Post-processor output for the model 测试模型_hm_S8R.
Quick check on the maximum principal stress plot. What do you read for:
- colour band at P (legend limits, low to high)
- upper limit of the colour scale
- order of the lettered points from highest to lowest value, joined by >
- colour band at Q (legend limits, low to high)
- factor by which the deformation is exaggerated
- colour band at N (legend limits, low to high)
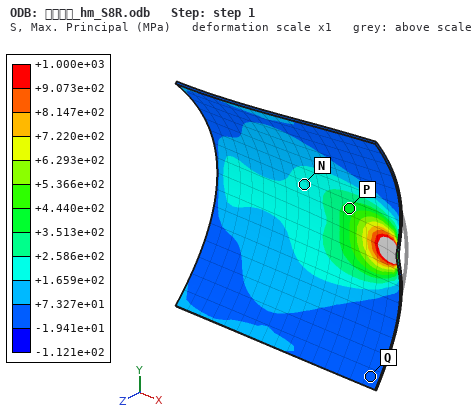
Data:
+3.513e+02 to +4.440e+02 MPa
+1.000e+03 MPa
P > N > Q
-1.941e+01 to +7.327e+01 MPa
1
+1.659e+02 to +2.586e+02 MPa
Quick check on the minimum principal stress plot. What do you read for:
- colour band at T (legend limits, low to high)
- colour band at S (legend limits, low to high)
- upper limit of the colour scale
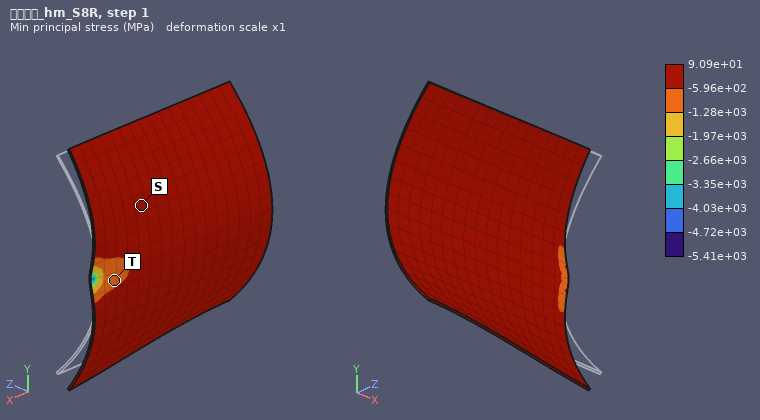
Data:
-1.28e+03 to -5.96e+02 MPa
-5.96e+02 to 9.09e+01 MPa
9.09e+01 MPa
